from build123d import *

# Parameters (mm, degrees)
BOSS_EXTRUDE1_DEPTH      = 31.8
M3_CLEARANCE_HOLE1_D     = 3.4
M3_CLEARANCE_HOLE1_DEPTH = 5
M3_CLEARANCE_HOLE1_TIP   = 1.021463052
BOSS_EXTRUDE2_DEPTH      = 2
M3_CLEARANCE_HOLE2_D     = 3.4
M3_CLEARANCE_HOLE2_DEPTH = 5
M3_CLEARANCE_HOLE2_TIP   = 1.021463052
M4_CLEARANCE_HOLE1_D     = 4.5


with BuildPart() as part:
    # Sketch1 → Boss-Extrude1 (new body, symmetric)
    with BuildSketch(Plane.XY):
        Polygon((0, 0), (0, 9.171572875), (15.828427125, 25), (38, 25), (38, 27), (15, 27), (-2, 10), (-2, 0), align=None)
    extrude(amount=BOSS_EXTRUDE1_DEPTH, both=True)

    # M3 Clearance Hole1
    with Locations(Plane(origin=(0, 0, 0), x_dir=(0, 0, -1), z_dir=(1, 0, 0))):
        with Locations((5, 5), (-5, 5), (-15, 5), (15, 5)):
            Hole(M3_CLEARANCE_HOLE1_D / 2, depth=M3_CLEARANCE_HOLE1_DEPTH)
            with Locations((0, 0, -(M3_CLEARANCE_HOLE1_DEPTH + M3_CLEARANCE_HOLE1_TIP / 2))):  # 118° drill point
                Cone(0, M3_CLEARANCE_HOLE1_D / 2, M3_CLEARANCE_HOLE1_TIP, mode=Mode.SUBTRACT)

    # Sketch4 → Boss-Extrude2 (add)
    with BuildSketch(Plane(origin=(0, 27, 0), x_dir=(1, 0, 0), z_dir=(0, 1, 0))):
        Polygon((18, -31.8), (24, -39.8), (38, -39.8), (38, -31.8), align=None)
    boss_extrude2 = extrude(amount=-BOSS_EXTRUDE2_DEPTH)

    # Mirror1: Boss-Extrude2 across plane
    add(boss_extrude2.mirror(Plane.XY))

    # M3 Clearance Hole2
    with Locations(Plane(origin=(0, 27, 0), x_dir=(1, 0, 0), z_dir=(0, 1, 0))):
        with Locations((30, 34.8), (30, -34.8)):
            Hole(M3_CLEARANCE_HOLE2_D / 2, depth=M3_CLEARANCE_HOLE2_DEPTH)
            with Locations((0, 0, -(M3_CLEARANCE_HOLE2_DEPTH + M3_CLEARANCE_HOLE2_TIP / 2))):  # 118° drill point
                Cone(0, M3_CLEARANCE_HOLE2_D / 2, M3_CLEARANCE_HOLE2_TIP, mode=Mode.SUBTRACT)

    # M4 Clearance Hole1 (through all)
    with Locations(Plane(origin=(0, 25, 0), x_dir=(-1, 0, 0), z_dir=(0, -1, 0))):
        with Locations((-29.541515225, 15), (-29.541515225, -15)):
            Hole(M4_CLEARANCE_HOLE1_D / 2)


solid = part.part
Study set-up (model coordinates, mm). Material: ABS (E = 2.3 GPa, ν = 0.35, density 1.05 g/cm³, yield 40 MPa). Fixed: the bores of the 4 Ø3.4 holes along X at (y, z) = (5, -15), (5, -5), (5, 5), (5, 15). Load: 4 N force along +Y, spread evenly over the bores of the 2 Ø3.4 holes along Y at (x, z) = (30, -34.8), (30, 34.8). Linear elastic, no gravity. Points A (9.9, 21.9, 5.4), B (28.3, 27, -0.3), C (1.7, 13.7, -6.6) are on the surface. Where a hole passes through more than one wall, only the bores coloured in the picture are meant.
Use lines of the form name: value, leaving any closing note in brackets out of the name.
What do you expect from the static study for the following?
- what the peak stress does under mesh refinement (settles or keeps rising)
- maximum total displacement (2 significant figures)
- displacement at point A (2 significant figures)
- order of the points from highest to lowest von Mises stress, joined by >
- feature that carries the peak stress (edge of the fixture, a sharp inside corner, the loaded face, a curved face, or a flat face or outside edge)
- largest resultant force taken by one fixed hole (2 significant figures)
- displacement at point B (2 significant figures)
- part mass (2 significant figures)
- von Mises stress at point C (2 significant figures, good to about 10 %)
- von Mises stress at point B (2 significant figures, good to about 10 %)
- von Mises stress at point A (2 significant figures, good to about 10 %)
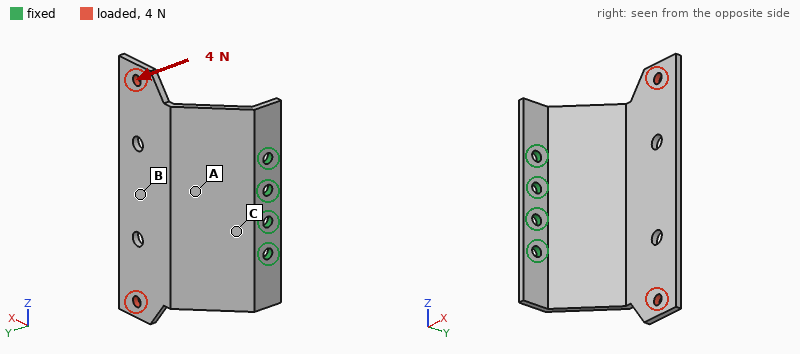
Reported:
what the peak stress does under mesh refinement: keeps rising
maximum total displacement: 1.1 mm
displacement at point A: 0.24 mm
order of the points from highest to lowest von Mises stress, joined by >: C > A > B
feature that carries the peak stress: edge of the fixture
largest resultant force taken by one fixed hole: 2.4 N
displacement at point B: 0.68 mm
part mass: 7.8 g
von Mises stress at point C: 2.6 MPa
von Mises stress at point B: 0.43 MPa
von Mises stress at point A: 1.5 MPa
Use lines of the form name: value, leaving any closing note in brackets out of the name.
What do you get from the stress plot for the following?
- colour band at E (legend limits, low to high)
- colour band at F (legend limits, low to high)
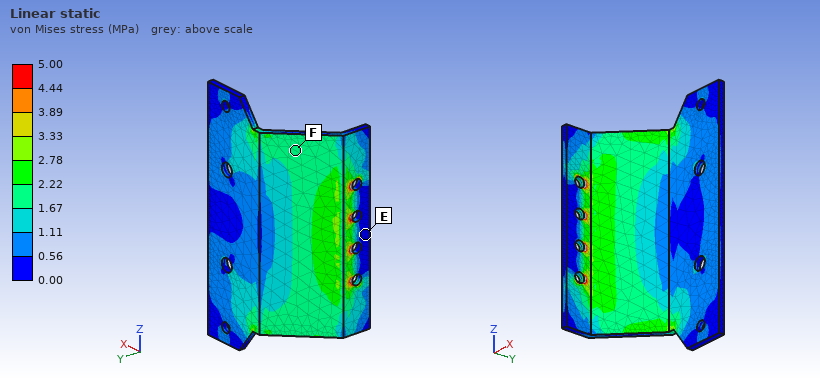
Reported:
colour band at E: 0.00 to 0.56 MPa
colour band at F: 1.67 to 2.22 MPa
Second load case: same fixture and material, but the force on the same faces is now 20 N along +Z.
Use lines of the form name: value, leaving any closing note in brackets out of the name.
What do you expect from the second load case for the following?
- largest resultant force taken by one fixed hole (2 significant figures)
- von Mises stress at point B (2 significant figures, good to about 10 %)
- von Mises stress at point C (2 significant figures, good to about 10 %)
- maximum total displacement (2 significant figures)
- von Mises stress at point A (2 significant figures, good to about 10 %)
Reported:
largest resultant force taken by one fixed hole: 22 N
von Mises stress at point B: 0.95 MPa
von Mises stress at point C: 1.6 MPa
maximum total displacement: 1.0 mm
von Mises stress at point A: 1.6 MPa
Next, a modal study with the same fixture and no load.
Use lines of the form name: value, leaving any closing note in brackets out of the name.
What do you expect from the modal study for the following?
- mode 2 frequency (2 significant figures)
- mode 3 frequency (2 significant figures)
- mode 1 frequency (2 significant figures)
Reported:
mode 2 frequency: 300 Hz
mode 3 frequency: 840 Hz
mode 1 frequency: 190 Hz
